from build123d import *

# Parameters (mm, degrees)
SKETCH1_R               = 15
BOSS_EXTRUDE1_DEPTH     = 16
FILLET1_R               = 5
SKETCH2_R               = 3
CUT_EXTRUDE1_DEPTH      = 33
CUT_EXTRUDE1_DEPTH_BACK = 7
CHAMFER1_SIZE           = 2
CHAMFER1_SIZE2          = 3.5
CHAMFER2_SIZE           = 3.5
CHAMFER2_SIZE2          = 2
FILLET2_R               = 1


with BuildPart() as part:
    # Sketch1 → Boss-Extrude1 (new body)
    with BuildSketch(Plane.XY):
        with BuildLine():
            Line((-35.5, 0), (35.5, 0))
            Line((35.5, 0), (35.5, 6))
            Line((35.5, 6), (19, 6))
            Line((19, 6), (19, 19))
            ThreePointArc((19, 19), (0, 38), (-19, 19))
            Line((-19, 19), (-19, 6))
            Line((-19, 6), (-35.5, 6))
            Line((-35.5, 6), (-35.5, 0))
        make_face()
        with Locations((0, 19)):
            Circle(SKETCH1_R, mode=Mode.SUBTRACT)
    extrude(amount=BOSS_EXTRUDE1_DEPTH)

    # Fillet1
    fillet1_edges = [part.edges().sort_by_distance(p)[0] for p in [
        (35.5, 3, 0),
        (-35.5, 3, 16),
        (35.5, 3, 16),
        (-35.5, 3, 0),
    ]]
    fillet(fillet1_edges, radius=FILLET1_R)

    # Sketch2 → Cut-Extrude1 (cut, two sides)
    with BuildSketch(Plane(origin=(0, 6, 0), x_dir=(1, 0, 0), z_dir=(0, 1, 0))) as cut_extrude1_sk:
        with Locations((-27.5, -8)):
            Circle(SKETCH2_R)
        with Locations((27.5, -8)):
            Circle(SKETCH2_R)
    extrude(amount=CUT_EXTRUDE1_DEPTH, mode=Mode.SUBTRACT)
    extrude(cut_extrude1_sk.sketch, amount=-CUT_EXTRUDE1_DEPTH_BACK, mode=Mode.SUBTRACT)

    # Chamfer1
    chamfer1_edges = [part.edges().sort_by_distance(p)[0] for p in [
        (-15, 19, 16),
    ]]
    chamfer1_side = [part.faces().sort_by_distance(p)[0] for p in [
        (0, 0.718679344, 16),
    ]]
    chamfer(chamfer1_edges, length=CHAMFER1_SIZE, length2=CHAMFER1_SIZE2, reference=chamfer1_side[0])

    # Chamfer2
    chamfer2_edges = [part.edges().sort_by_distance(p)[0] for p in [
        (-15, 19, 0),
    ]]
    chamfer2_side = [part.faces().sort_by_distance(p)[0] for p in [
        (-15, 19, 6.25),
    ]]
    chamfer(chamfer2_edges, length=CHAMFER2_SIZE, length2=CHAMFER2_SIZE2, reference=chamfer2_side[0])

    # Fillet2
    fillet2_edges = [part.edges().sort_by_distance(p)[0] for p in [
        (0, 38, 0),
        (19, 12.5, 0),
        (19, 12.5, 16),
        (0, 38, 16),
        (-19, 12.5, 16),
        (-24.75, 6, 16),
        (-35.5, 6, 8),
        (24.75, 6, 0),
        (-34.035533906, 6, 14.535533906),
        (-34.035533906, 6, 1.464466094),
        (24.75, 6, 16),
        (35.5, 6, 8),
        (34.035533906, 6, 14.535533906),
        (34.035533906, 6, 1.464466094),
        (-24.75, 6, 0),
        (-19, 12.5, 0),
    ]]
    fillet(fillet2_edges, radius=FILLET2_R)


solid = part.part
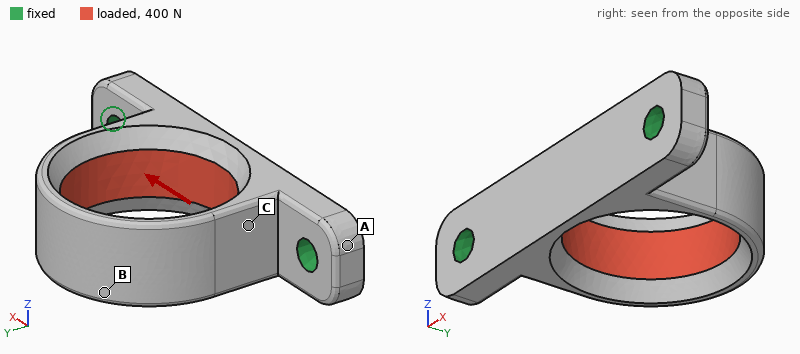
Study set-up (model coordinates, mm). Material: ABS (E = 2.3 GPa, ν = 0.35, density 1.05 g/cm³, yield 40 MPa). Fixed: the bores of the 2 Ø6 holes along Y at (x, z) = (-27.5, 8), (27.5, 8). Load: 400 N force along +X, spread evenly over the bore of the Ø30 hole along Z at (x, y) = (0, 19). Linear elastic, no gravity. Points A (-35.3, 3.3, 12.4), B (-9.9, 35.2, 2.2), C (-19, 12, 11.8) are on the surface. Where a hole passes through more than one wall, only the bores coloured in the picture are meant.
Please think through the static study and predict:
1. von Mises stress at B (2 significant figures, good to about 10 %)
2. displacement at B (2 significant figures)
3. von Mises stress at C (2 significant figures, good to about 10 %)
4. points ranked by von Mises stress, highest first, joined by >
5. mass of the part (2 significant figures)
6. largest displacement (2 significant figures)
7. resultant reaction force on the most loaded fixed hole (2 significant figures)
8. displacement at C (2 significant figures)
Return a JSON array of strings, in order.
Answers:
["9.2 MPa", "0.61 mm", "14 MPa", "C > B > A", "12 g", "0.62 mm", "240 N", "0.10 mm"]
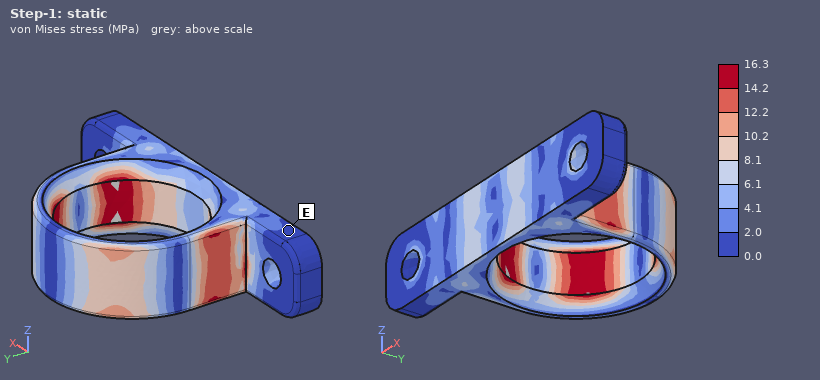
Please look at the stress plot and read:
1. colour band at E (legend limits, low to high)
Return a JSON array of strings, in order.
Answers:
["0.0 to 2.0 MPa"]
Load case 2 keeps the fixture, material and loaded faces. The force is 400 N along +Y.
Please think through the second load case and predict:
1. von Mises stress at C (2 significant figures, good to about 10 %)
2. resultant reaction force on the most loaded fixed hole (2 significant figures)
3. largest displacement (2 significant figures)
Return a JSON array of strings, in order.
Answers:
["7.2 MPa", "200 N", "0.18 mm"]
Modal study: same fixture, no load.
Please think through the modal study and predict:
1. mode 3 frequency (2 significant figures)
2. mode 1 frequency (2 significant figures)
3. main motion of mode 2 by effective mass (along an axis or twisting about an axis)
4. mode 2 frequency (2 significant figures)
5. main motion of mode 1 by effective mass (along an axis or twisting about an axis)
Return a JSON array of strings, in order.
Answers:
["2700 Hz", "1200 Hz", "along X", "1700 Hz", "along Z"]
